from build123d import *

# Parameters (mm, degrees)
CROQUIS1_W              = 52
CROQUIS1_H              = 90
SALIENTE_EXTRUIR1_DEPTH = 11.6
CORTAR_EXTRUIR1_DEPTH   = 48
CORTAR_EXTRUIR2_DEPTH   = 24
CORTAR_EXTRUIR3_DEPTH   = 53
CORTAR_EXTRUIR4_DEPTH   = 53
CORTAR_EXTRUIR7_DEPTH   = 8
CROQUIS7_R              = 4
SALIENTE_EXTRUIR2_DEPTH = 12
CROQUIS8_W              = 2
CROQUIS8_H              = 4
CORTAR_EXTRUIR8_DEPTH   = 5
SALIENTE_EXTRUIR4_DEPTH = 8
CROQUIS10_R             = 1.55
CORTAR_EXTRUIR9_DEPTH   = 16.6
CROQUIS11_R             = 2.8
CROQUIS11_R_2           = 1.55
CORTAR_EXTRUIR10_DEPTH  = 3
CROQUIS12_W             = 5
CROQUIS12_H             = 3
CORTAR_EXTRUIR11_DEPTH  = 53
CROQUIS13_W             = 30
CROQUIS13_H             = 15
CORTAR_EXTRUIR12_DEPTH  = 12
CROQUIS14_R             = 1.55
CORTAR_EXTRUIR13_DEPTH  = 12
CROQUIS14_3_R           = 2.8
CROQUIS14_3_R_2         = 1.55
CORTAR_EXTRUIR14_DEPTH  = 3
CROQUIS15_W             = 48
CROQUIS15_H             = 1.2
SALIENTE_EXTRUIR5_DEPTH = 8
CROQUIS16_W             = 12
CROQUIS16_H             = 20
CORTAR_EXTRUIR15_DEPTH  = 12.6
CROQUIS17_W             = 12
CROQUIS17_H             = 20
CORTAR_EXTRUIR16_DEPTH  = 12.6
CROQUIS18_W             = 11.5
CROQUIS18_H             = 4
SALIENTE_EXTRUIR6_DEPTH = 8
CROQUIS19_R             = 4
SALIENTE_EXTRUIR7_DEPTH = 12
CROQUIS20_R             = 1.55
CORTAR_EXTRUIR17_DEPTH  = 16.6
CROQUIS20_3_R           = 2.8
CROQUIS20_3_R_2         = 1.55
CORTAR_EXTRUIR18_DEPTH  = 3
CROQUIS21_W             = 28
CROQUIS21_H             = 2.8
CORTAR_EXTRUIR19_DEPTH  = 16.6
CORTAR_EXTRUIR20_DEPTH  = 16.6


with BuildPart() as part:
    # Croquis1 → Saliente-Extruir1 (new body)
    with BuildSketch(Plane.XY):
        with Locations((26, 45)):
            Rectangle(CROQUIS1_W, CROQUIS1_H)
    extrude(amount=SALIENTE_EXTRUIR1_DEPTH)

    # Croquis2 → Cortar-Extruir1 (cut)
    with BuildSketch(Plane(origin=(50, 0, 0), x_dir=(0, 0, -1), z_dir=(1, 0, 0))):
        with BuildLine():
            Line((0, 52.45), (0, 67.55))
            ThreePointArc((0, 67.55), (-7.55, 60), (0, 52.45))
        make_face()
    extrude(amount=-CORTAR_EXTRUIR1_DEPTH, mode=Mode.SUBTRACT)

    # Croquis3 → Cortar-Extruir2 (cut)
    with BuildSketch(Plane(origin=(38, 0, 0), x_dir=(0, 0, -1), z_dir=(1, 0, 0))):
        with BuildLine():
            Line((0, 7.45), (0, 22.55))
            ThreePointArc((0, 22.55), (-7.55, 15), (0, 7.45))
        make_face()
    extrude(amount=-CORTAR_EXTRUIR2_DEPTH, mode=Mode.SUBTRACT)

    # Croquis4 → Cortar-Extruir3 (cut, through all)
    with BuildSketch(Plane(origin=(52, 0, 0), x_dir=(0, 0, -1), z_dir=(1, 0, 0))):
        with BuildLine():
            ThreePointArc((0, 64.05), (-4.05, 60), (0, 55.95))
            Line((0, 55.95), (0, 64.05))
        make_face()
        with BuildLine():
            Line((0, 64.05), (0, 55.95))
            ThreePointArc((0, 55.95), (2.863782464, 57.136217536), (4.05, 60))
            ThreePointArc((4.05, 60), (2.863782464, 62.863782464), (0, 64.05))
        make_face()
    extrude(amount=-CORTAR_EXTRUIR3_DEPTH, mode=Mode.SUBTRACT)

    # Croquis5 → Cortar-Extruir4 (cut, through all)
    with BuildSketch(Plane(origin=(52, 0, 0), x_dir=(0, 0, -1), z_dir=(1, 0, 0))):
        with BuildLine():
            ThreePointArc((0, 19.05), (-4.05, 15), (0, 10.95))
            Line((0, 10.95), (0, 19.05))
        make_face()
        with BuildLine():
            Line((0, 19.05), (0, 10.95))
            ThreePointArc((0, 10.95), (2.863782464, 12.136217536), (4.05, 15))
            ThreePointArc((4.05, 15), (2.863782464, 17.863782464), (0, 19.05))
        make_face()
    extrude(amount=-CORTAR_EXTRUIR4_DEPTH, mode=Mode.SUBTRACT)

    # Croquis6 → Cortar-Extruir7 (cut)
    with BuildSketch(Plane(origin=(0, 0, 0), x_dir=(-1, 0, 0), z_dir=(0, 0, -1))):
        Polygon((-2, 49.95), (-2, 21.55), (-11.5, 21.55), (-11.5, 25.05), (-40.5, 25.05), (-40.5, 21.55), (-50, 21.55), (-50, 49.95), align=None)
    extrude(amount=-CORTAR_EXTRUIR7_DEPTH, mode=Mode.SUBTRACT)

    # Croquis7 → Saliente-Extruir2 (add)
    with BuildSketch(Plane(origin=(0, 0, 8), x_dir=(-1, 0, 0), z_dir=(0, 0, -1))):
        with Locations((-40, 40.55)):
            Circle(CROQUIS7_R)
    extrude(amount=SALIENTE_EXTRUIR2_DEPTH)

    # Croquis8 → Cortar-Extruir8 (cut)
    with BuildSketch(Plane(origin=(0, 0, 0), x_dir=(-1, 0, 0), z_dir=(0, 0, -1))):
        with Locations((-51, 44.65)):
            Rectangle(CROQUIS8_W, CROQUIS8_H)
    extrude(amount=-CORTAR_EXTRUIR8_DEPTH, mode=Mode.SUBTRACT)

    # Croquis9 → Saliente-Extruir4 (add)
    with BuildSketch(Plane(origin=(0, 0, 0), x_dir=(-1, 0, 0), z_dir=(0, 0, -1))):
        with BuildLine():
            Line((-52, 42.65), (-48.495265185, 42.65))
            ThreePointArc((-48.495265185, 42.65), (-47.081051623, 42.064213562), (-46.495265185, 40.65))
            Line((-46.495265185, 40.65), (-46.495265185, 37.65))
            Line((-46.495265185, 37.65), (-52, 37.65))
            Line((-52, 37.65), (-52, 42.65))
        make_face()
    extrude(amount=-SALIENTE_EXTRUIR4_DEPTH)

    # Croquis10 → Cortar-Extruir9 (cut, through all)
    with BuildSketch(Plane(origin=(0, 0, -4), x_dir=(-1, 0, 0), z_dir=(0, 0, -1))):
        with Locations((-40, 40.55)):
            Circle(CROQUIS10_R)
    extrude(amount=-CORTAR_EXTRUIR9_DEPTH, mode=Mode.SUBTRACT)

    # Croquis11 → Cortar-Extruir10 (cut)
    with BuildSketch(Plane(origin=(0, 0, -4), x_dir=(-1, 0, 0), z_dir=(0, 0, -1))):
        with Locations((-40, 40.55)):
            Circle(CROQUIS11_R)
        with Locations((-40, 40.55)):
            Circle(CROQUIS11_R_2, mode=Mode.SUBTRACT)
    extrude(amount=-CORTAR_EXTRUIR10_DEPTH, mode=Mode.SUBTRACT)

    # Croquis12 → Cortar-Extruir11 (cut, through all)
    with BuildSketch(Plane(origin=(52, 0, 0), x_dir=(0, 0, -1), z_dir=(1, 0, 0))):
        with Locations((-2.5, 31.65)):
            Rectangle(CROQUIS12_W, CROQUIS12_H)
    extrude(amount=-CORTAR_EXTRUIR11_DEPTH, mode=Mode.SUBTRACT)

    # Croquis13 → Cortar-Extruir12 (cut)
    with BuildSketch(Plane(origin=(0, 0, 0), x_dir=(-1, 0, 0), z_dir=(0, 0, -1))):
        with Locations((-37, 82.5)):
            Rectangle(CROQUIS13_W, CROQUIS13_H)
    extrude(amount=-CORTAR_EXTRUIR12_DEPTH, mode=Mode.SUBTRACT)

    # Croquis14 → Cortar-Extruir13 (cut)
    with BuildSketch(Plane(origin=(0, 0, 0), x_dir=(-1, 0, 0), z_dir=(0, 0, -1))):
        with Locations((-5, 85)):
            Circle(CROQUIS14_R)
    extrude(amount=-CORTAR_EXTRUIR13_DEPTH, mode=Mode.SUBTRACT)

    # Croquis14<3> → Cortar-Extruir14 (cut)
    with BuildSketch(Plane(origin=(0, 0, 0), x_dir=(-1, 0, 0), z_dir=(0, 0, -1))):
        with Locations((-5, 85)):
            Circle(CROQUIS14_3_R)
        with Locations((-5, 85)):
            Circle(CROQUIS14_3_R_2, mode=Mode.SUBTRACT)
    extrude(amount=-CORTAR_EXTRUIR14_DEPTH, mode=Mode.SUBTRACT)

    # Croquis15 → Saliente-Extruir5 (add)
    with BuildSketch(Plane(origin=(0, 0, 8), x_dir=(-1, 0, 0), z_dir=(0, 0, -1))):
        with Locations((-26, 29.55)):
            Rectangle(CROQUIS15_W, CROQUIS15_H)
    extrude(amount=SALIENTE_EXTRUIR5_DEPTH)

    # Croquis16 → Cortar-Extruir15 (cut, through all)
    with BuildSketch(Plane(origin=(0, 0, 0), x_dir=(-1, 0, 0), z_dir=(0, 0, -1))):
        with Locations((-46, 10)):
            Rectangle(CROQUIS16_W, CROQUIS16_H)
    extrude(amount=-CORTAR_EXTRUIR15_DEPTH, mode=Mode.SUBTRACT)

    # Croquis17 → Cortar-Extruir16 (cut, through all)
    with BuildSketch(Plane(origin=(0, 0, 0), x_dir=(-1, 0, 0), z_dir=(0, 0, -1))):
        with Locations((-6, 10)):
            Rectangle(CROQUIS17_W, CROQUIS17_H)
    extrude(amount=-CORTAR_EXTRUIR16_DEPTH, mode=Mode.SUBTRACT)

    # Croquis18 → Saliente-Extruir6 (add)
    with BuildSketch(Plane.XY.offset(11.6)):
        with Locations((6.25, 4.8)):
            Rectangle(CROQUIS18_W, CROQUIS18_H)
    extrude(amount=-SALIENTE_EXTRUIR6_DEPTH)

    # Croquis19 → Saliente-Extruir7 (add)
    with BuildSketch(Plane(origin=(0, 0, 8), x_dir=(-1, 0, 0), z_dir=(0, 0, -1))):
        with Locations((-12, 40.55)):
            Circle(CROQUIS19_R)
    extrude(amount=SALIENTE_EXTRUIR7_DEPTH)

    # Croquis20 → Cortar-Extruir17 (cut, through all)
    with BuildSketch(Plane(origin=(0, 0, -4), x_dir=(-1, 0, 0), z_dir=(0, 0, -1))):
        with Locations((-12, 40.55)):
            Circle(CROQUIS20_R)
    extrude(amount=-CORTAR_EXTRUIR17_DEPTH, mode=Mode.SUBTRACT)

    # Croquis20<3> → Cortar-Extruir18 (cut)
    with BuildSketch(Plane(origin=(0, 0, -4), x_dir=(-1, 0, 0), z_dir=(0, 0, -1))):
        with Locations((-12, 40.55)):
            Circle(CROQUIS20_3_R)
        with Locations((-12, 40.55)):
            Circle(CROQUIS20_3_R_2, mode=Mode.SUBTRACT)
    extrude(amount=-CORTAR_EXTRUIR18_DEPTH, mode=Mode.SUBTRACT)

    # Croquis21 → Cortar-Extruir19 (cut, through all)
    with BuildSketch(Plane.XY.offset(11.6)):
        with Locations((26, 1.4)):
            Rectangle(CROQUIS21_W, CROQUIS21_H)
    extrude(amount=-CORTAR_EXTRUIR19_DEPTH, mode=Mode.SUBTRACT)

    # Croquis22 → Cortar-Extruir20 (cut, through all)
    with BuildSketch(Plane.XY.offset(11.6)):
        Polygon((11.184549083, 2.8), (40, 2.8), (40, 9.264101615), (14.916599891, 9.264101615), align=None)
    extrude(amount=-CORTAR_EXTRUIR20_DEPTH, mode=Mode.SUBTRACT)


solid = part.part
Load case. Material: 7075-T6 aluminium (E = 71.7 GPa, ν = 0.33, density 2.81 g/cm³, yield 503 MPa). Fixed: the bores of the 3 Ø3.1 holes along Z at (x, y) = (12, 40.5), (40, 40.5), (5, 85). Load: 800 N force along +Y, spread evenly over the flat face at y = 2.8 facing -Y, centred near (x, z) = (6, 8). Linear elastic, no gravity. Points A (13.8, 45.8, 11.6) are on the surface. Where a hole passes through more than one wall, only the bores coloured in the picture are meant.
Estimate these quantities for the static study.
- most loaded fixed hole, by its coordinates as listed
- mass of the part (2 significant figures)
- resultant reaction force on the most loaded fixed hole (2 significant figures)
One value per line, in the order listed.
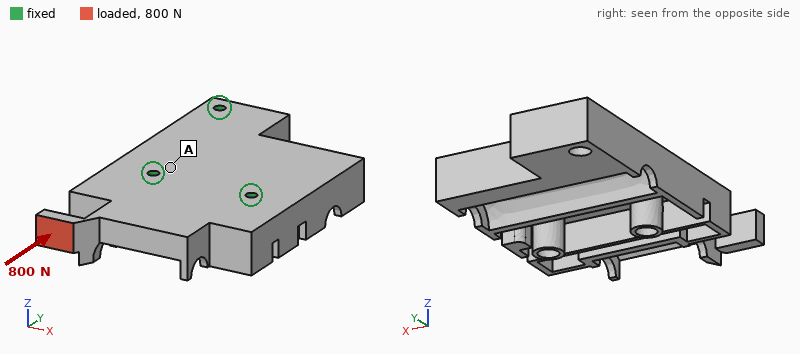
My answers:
(12, 40.5)
72 g
750 N
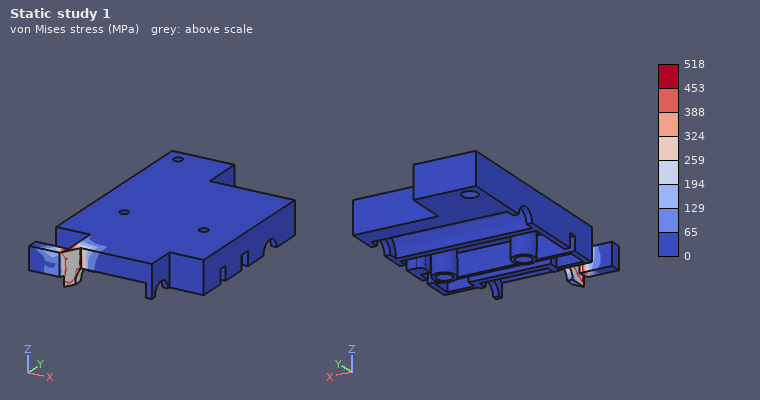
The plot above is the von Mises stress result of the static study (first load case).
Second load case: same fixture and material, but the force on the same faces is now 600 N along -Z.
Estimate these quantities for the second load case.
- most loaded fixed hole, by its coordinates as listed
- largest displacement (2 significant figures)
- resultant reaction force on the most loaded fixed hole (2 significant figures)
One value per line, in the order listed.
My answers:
(12, 40.5)
0.96 mm
940 N
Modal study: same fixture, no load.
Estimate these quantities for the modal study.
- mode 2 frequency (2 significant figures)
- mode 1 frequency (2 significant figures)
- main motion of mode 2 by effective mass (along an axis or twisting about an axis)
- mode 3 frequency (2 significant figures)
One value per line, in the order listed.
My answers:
4900 Hz
2900 Hz
along Z
5200 Hz
